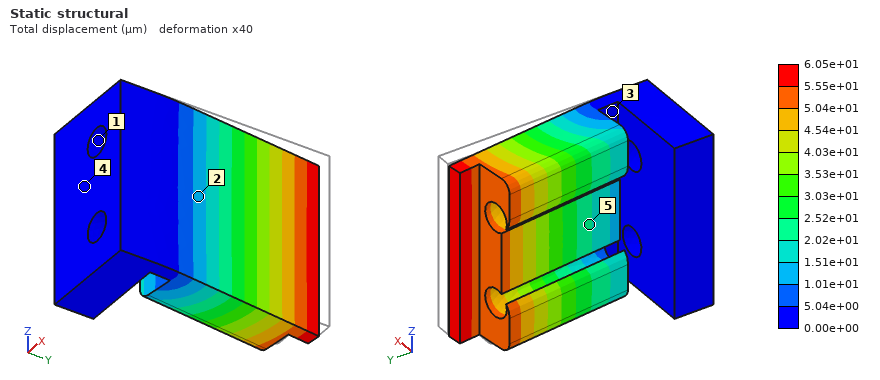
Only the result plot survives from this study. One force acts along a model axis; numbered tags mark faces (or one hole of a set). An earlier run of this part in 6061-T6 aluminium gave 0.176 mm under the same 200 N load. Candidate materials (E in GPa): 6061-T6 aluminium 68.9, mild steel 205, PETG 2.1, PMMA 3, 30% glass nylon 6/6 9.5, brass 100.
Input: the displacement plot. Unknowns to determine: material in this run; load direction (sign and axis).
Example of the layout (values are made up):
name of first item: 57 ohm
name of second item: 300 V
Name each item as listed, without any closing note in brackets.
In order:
material in this run: mild steel
load direction: -X
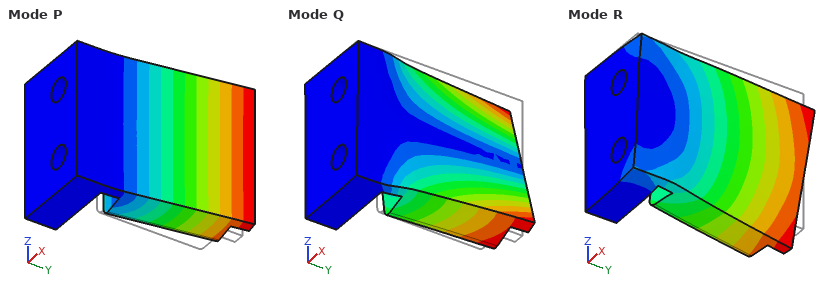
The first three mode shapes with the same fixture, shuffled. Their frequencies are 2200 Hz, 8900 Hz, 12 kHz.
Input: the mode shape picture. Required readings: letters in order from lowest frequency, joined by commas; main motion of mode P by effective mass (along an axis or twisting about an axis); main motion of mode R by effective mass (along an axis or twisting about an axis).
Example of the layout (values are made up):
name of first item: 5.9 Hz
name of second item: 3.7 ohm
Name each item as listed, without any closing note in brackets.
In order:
letters in order from lowest frequency, joined by commas: P, Q, R
main motion of mode P by effective mass: along X
main motion of mode R by effective mass: along Z
